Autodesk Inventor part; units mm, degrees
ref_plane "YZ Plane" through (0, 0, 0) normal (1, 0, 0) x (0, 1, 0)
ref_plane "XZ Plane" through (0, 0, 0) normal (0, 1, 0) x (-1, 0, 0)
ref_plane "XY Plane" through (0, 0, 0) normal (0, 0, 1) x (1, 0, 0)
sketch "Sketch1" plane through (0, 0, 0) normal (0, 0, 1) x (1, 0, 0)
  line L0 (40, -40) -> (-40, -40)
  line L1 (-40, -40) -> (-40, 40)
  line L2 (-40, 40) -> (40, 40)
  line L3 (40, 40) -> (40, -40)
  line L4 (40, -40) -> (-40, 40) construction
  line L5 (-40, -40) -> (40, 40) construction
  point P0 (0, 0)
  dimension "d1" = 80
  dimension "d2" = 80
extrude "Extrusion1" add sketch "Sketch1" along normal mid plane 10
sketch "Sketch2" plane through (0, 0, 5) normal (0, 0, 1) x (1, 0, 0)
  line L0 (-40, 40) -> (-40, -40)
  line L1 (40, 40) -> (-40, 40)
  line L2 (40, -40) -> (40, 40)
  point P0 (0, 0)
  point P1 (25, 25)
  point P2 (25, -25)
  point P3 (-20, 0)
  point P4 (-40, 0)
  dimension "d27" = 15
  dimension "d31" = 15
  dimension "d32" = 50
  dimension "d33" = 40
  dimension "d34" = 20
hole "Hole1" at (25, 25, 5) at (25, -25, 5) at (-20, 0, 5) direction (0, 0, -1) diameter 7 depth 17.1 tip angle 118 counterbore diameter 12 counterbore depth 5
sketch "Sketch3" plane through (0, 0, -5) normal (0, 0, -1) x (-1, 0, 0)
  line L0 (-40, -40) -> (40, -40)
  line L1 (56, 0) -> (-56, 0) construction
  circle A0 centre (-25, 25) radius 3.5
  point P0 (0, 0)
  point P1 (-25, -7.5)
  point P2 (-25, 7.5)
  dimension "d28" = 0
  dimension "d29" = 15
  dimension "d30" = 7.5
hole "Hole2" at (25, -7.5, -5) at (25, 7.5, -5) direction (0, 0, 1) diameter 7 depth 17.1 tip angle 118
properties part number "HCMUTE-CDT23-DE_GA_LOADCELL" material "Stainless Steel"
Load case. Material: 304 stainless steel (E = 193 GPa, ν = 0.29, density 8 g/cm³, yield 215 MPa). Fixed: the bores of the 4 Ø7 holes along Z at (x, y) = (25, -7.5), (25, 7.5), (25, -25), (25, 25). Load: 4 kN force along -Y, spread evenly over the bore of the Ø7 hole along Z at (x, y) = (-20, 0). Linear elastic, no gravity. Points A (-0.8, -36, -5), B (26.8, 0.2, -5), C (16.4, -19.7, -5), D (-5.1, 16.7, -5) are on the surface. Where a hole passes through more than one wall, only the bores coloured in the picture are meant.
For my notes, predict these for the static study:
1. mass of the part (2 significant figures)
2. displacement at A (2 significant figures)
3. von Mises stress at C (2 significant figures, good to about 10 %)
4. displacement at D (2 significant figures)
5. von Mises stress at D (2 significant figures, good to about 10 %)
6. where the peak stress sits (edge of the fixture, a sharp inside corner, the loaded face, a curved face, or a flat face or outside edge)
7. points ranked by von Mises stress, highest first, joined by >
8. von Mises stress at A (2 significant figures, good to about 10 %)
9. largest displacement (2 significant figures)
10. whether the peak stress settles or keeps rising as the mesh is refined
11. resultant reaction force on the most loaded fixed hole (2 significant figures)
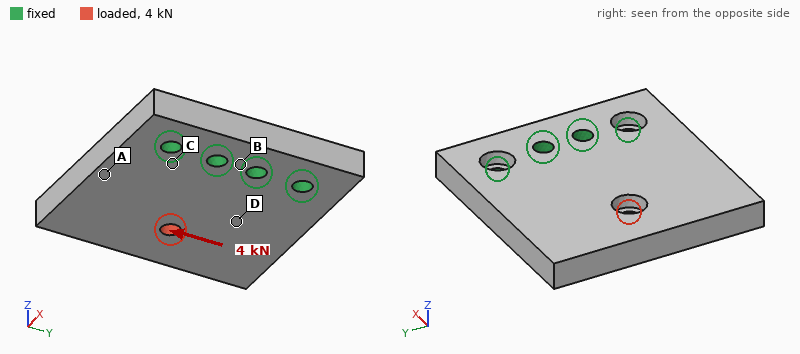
490 g
7.0 µm
27 MPa
5.9 µm
17 MPa
edge of the fixture
C > D > A > B
9.5 MPa
15 µm
keeps rising
3.0 kN
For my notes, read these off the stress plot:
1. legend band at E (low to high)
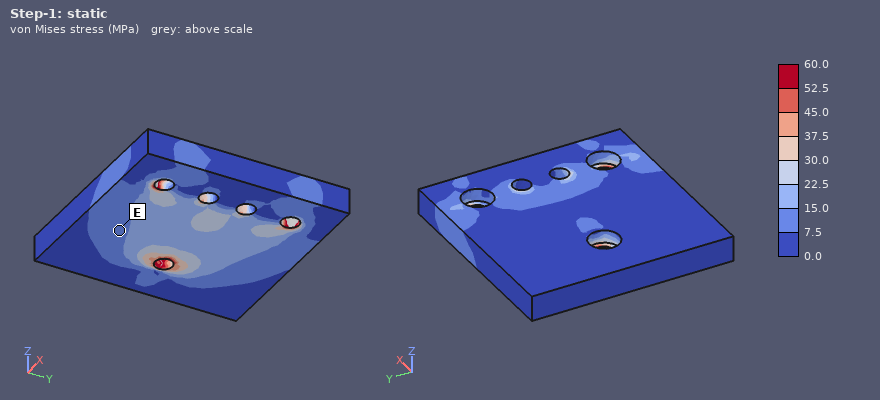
7.5 to 15.0 MPa
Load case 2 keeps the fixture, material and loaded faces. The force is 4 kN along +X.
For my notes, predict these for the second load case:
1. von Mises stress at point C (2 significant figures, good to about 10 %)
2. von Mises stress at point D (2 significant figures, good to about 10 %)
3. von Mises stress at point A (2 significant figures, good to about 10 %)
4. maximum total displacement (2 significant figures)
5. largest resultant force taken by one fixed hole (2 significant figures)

13 MPa
13 MPa
7.5 MPa
15 µm
1.0 kN
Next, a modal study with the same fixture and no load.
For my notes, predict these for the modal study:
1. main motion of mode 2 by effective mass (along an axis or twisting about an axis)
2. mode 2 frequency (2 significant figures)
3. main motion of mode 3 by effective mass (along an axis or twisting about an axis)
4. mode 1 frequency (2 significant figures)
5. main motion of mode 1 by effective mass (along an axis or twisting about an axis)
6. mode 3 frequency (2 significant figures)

twisting about X
3300 Hz
along Y
1800 Hz
along Z
7000 Hz
